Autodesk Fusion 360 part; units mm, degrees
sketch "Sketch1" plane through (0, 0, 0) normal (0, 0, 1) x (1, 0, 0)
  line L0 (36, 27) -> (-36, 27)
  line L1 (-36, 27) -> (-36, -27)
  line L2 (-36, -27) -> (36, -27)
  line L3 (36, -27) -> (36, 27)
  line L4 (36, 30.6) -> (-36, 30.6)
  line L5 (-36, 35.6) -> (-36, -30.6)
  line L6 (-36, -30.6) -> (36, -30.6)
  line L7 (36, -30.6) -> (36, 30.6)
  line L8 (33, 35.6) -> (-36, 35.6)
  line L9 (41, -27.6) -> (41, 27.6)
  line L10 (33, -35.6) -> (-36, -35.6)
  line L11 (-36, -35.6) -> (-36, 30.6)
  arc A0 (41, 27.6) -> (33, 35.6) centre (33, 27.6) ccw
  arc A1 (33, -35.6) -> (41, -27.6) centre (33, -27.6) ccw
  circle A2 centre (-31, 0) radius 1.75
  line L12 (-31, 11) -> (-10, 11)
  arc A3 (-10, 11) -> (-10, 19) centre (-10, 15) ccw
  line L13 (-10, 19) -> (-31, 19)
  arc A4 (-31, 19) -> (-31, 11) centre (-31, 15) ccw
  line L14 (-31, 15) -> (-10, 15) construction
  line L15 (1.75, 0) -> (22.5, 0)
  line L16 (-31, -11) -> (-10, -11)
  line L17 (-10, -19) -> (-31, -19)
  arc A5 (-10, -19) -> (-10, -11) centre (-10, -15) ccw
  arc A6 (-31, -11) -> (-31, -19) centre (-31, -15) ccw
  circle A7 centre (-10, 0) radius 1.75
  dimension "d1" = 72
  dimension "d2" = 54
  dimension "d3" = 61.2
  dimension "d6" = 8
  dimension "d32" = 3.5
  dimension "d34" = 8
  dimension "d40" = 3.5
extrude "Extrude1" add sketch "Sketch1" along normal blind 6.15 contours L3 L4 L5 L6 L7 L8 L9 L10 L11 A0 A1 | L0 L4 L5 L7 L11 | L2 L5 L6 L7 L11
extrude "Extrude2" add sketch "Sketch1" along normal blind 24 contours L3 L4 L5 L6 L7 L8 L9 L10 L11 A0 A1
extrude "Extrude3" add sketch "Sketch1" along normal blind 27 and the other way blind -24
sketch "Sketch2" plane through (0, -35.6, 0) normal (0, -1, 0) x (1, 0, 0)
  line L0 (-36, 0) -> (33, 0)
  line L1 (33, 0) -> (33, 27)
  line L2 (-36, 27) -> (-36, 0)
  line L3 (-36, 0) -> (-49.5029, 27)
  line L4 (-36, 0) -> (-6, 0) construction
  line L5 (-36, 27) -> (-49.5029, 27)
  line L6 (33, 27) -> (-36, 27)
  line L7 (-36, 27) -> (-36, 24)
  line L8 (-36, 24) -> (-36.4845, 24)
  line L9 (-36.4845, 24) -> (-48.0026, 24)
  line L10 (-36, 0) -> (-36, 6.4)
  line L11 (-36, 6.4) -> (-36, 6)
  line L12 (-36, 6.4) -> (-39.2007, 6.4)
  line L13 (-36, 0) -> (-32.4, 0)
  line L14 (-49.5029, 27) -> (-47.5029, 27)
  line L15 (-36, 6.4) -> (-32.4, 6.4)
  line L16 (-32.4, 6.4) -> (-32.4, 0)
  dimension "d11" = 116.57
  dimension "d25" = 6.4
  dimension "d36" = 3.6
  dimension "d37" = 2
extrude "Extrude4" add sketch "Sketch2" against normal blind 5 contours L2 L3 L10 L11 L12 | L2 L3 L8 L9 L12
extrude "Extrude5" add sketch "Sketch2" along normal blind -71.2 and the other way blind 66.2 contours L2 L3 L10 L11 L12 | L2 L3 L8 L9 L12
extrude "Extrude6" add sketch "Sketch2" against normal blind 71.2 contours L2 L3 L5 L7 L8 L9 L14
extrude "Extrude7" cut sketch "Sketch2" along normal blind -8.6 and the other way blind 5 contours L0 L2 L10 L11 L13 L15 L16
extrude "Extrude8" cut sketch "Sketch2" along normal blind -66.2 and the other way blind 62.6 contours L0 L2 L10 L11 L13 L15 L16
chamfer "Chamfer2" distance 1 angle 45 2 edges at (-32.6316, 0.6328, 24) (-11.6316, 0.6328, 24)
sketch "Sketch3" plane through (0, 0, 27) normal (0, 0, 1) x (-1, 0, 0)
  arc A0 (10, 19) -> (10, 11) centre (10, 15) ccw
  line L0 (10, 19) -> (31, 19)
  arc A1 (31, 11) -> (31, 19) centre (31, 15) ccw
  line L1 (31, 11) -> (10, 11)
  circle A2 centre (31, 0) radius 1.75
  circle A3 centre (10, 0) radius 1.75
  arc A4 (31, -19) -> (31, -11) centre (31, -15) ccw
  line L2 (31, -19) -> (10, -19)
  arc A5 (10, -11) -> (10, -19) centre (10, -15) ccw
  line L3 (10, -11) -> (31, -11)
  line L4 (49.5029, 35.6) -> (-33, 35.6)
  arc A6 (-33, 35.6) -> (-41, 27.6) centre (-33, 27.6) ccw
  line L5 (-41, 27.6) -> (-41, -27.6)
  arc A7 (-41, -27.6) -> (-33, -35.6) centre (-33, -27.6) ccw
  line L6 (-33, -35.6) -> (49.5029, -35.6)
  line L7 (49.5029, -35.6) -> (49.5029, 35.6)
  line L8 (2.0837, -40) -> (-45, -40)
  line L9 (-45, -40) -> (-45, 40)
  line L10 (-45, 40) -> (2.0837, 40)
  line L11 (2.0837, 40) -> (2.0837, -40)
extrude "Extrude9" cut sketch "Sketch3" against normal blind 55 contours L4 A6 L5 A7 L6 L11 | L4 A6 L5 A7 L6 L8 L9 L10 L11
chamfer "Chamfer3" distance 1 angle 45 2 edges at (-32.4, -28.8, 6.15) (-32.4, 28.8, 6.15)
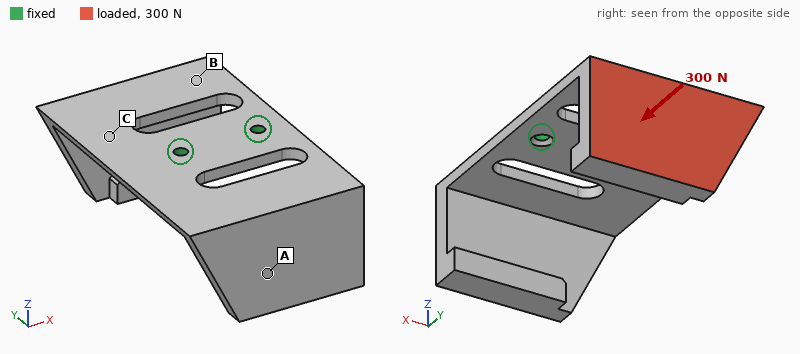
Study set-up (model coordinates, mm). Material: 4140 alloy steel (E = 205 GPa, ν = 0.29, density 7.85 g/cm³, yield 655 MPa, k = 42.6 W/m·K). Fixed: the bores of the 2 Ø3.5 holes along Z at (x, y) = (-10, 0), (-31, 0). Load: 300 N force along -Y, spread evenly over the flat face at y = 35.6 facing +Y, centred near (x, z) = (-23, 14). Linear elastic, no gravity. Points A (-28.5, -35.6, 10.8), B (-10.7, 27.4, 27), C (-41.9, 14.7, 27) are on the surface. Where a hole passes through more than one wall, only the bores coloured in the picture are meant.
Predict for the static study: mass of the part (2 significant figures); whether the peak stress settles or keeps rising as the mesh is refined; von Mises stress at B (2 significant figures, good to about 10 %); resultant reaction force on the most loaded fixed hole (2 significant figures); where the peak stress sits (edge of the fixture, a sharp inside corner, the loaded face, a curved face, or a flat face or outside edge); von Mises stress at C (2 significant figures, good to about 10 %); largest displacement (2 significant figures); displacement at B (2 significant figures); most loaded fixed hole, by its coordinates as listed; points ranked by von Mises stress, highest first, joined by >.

150 g
keeps rising
34 MPa
170 N
edge of the fixture
100 MPa
0.33 mm
0.12 mm
(-31, 0)
C > B > A
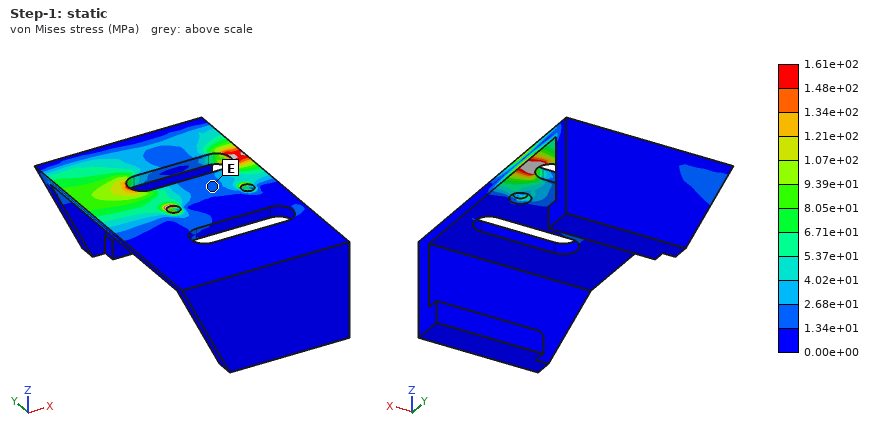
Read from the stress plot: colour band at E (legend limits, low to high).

1.34e+01 to 2.68e+01 MPa
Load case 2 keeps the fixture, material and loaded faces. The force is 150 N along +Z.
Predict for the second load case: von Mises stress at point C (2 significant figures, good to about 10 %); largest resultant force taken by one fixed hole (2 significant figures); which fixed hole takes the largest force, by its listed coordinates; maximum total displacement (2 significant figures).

95 MPa
85 N
(-31, 0)
0.32 mm
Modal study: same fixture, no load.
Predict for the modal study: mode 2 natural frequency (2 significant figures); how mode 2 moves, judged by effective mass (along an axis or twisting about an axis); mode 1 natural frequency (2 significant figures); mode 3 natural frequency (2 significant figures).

570 Hz
along Z
500 Hz
1300 Hz
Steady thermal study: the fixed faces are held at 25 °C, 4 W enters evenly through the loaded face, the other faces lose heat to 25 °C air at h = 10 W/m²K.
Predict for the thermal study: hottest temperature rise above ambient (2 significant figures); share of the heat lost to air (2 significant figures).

37 K
32 %
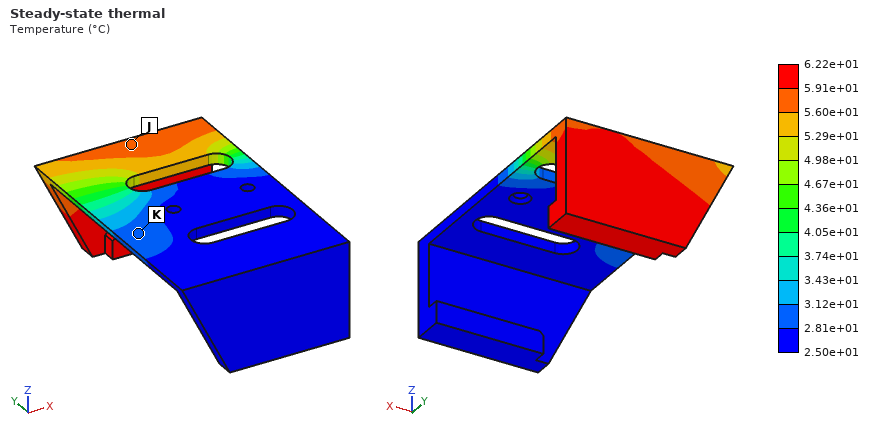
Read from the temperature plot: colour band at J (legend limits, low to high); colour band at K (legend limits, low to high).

5.60e+01 to 5.91e+01 °C
2.81e+01 to 3.12e+01 °C
